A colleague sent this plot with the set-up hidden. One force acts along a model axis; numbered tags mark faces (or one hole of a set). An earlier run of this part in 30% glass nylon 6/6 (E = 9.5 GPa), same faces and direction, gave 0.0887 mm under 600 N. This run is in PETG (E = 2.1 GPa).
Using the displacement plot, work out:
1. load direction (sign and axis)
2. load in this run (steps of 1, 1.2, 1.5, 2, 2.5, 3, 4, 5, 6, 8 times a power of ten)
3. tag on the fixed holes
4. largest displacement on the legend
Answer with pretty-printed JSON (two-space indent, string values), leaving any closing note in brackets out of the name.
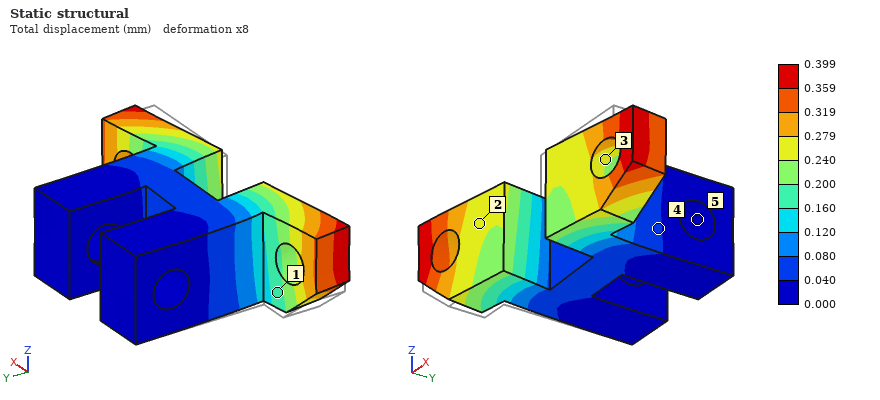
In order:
{
  "load direction": "+X",
  "load in this run": "600 N",
  "tag on the fixed holes": "5",
  "largest displacement on the legend": "0.399 mm"
}
